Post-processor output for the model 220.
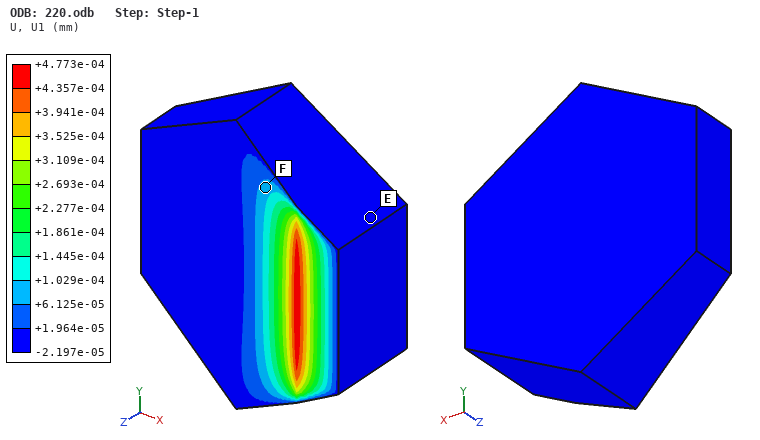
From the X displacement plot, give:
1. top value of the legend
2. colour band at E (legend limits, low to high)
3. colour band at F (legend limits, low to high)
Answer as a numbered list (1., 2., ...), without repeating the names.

1. +4.773e-04 mm
2. -2.197e-05 to +1.964e-05 mm
3. +6.125e-05 to +1.029e-04 mm
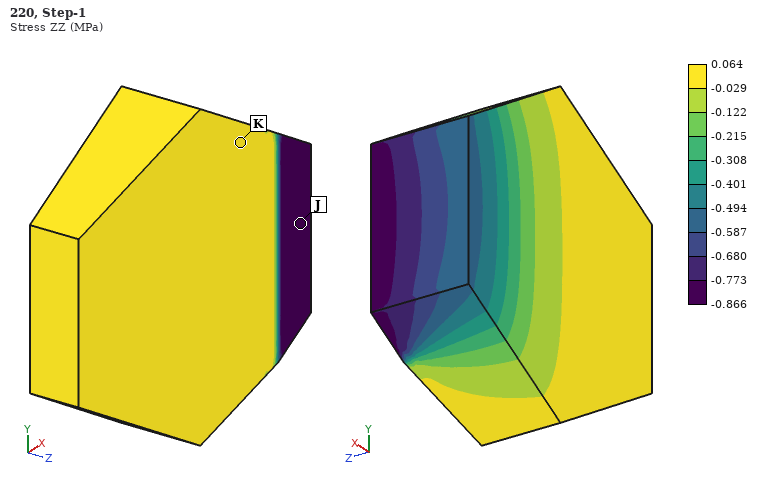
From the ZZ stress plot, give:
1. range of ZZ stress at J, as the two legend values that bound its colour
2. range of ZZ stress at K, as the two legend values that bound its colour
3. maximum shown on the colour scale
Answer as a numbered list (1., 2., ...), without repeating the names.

1. -0.866 to -0.773 MPa
2. -0.029 to 0.064 MPa
3. 0.064 MPa
